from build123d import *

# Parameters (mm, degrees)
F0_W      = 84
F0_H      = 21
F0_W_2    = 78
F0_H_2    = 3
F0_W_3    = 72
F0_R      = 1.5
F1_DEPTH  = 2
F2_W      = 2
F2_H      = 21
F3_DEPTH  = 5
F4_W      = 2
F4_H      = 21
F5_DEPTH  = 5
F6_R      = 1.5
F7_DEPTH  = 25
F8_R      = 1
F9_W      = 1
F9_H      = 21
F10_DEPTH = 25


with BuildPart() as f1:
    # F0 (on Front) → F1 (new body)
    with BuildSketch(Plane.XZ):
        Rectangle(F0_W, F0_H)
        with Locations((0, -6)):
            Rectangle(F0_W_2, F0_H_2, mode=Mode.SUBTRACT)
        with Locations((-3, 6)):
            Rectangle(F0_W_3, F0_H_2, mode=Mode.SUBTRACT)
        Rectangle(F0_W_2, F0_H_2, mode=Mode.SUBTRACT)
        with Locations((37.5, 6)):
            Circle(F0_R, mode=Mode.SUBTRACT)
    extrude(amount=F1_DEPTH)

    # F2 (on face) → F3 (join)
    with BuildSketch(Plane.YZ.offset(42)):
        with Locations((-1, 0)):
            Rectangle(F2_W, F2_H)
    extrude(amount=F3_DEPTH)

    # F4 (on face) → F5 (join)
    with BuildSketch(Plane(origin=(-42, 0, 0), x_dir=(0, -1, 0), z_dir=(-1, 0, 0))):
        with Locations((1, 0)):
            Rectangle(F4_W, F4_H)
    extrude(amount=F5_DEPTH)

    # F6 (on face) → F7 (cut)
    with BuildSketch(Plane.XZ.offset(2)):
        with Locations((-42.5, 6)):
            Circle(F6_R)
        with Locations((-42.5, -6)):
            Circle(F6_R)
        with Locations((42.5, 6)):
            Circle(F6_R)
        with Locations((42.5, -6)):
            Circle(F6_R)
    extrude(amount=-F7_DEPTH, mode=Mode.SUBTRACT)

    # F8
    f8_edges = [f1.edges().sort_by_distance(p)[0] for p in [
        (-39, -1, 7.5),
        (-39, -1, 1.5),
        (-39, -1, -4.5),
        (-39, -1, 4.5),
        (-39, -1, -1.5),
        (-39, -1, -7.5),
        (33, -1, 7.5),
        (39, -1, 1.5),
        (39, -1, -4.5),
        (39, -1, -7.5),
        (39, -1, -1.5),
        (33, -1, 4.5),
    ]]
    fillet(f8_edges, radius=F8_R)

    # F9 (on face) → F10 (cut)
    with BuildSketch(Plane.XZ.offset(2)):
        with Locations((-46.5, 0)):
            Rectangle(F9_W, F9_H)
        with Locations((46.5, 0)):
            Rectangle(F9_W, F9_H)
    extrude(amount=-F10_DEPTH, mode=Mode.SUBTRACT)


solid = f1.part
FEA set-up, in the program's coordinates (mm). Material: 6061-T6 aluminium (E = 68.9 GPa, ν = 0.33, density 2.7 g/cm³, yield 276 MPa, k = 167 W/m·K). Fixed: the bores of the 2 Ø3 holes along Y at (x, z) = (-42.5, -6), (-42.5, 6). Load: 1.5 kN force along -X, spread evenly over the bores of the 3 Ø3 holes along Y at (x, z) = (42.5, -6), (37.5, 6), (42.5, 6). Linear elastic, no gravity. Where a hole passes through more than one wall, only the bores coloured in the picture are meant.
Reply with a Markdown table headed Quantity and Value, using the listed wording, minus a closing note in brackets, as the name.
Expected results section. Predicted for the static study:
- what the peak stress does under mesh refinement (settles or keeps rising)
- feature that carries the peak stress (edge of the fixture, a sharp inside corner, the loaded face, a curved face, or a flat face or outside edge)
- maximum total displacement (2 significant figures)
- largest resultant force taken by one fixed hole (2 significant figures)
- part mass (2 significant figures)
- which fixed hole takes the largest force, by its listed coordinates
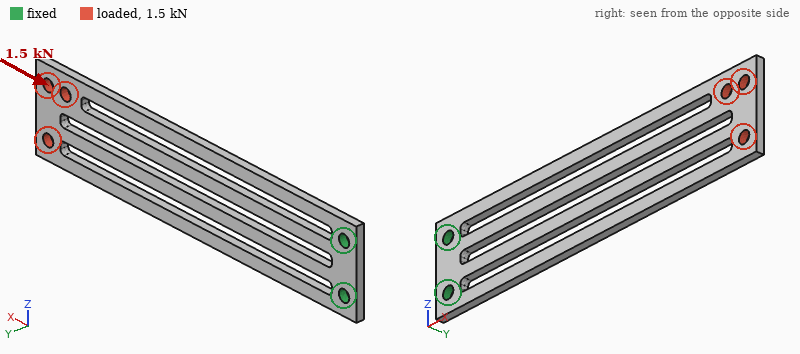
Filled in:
| Quantity | Value |
|---|---|
| what the peak stress does under mesh refinement | keeps rising |
| feature that carries the peak stress | edge of the fixture |
| maximum total displacement | 0.19 mm |
| largest resultant force taken by one fixed hole | 950 N |
| part mass | 6.6 g |
| which fixed hole takes the largest force, by its listed coordinates | (-42.5, 6) |
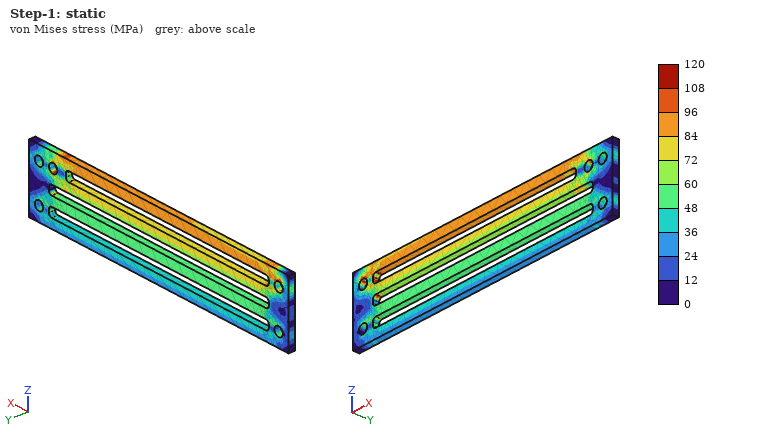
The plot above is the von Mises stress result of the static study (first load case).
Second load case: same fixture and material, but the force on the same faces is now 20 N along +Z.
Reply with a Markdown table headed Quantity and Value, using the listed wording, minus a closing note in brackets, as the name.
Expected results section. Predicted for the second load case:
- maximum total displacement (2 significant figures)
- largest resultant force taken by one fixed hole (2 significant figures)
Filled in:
| Quantity | Value |
|---|---|
| maximum total displacement | 0.66 mm |
| largest resultant force taken by one fixed hole | 100 N |
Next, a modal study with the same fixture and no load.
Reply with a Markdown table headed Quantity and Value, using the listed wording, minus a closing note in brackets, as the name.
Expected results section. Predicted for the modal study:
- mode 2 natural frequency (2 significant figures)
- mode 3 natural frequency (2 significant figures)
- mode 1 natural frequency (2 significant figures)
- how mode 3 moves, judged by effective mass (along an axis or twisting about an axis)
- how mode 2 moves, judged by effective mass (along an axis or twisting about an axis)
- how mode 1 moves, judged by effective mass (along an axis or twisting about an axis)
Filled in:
| Quantity | Value |
|---|---|
| mode 2 natural frequency | 530 Hz |
| mode 3 natural frequency | 1100 Hz |
| mode 1 natural frequency | 200 Hz |
| how mode 3 moves, judged by effective mass | twisting about X |
| how mode 2 moves, judged by effective mass | along Z |
| how mode 1 moves, judged by effective mass | along Y |
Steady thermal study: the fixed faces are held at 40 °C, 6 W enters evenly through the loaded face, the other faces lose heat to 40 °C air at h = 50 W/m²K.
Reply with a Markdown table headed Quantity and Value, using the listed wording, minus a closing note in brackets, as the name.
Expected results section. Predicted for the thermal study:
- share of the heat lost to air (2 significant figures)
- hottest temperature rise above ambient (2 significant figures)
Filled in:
| Quantity | Value |
|---|---|
| share of the heat lost to air | 73 % |
| hottest temperature rise above ambient | 57 K |
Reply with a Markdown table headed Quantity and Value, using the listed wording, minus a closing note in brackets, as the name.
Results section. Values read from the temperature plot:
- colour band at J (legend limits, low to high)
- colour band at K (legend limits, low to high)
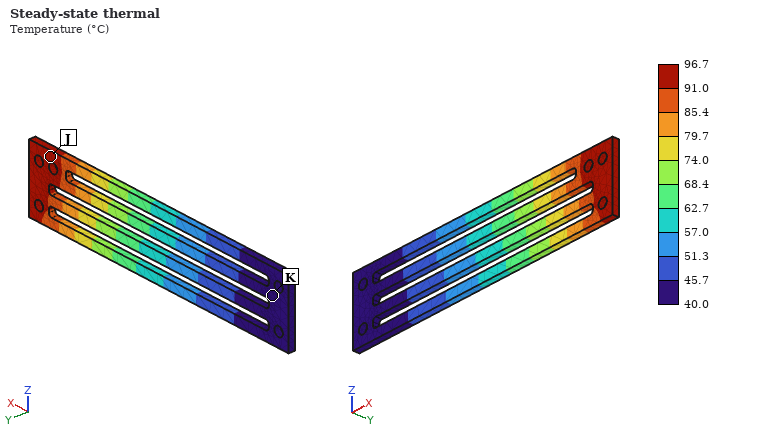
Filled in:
| Quantity | Value |
|---|---|
| colour band at J | 91.0 to 96.7 °C |
| colour band at K | 40.0 to 45.7 °C |
